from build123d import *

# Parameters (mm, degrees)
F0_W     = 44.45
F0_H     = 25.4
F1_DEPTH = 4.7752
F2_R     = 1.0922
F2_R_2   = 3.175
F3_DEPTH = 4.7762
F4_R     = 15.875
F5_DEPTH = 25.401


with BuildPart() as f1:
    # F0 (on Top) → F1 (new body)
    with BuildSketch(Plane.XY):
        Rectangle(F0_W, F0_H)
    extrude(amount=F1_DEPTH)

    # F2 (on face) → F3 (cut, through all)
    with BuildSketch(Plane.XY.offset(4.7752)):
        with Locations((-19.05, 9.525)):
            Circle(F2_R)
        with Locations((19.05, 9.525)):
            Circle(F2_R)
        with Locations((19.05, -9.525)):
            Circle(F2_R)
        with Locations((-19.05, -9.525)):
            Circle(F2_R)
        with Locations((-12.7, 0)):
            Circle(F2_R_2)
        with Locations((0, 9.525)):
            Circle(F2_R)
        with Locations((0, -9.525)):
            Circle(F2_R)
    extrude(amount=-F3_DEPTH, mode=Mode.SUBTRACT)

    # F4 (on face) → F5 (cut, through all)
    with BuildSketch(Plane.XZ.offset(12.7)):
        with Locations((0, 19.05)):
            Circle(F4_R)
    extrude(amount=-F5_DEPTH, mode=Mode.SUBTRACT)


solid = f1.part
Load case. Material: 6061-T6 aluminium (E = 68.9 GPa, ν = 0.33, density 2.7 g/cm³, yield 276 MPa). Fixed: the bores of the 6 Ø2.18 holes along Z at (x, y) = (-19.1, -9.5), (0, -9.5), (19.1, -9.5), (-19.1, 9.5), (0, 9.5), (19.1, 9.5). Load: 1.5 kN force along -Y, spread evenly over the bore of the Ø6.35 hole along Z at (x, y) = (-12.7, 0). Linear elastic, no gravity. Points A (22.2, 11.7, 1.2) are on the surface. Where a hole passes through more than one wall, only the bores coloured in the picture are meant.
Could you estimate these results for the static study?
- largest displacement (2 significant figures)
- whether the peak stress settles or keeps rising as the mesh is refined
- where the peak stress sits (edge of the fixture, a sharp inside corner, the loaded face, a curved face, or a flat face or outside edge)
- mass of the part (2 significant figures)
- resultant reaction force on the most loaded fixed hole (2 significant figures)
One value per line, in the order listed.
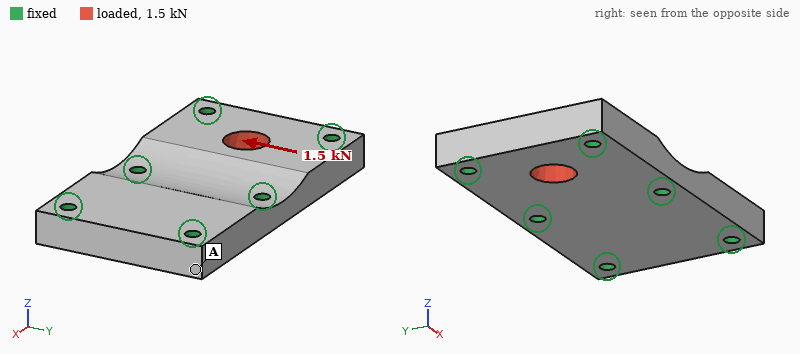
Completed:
3.2 µm
keeps rising
edge of the fixture
13 g
510 N
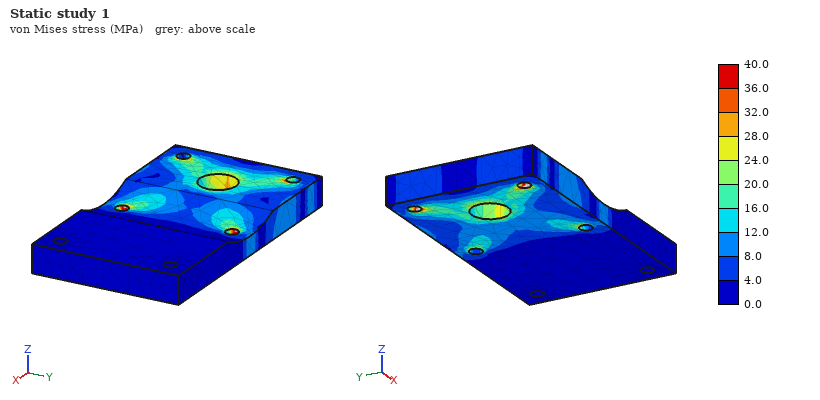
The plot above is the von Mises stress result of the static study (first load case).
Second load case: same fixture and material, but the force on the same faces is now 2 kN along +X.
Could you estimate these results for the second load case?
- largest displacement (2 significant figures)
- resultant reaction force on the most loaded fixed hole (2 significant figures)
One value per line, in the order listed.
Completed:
5.5 µm
590 N
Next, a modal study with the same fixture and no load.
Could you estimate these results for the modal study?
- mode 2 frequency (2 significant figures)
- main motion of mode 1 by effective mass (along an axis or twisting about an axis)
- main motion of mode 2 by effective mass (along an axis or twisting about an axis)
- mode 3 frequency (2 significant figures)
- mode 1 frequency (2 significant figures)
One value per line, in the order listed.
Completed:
37 kHz
along Z
twisting about Y
49 kHz
33 kHz
